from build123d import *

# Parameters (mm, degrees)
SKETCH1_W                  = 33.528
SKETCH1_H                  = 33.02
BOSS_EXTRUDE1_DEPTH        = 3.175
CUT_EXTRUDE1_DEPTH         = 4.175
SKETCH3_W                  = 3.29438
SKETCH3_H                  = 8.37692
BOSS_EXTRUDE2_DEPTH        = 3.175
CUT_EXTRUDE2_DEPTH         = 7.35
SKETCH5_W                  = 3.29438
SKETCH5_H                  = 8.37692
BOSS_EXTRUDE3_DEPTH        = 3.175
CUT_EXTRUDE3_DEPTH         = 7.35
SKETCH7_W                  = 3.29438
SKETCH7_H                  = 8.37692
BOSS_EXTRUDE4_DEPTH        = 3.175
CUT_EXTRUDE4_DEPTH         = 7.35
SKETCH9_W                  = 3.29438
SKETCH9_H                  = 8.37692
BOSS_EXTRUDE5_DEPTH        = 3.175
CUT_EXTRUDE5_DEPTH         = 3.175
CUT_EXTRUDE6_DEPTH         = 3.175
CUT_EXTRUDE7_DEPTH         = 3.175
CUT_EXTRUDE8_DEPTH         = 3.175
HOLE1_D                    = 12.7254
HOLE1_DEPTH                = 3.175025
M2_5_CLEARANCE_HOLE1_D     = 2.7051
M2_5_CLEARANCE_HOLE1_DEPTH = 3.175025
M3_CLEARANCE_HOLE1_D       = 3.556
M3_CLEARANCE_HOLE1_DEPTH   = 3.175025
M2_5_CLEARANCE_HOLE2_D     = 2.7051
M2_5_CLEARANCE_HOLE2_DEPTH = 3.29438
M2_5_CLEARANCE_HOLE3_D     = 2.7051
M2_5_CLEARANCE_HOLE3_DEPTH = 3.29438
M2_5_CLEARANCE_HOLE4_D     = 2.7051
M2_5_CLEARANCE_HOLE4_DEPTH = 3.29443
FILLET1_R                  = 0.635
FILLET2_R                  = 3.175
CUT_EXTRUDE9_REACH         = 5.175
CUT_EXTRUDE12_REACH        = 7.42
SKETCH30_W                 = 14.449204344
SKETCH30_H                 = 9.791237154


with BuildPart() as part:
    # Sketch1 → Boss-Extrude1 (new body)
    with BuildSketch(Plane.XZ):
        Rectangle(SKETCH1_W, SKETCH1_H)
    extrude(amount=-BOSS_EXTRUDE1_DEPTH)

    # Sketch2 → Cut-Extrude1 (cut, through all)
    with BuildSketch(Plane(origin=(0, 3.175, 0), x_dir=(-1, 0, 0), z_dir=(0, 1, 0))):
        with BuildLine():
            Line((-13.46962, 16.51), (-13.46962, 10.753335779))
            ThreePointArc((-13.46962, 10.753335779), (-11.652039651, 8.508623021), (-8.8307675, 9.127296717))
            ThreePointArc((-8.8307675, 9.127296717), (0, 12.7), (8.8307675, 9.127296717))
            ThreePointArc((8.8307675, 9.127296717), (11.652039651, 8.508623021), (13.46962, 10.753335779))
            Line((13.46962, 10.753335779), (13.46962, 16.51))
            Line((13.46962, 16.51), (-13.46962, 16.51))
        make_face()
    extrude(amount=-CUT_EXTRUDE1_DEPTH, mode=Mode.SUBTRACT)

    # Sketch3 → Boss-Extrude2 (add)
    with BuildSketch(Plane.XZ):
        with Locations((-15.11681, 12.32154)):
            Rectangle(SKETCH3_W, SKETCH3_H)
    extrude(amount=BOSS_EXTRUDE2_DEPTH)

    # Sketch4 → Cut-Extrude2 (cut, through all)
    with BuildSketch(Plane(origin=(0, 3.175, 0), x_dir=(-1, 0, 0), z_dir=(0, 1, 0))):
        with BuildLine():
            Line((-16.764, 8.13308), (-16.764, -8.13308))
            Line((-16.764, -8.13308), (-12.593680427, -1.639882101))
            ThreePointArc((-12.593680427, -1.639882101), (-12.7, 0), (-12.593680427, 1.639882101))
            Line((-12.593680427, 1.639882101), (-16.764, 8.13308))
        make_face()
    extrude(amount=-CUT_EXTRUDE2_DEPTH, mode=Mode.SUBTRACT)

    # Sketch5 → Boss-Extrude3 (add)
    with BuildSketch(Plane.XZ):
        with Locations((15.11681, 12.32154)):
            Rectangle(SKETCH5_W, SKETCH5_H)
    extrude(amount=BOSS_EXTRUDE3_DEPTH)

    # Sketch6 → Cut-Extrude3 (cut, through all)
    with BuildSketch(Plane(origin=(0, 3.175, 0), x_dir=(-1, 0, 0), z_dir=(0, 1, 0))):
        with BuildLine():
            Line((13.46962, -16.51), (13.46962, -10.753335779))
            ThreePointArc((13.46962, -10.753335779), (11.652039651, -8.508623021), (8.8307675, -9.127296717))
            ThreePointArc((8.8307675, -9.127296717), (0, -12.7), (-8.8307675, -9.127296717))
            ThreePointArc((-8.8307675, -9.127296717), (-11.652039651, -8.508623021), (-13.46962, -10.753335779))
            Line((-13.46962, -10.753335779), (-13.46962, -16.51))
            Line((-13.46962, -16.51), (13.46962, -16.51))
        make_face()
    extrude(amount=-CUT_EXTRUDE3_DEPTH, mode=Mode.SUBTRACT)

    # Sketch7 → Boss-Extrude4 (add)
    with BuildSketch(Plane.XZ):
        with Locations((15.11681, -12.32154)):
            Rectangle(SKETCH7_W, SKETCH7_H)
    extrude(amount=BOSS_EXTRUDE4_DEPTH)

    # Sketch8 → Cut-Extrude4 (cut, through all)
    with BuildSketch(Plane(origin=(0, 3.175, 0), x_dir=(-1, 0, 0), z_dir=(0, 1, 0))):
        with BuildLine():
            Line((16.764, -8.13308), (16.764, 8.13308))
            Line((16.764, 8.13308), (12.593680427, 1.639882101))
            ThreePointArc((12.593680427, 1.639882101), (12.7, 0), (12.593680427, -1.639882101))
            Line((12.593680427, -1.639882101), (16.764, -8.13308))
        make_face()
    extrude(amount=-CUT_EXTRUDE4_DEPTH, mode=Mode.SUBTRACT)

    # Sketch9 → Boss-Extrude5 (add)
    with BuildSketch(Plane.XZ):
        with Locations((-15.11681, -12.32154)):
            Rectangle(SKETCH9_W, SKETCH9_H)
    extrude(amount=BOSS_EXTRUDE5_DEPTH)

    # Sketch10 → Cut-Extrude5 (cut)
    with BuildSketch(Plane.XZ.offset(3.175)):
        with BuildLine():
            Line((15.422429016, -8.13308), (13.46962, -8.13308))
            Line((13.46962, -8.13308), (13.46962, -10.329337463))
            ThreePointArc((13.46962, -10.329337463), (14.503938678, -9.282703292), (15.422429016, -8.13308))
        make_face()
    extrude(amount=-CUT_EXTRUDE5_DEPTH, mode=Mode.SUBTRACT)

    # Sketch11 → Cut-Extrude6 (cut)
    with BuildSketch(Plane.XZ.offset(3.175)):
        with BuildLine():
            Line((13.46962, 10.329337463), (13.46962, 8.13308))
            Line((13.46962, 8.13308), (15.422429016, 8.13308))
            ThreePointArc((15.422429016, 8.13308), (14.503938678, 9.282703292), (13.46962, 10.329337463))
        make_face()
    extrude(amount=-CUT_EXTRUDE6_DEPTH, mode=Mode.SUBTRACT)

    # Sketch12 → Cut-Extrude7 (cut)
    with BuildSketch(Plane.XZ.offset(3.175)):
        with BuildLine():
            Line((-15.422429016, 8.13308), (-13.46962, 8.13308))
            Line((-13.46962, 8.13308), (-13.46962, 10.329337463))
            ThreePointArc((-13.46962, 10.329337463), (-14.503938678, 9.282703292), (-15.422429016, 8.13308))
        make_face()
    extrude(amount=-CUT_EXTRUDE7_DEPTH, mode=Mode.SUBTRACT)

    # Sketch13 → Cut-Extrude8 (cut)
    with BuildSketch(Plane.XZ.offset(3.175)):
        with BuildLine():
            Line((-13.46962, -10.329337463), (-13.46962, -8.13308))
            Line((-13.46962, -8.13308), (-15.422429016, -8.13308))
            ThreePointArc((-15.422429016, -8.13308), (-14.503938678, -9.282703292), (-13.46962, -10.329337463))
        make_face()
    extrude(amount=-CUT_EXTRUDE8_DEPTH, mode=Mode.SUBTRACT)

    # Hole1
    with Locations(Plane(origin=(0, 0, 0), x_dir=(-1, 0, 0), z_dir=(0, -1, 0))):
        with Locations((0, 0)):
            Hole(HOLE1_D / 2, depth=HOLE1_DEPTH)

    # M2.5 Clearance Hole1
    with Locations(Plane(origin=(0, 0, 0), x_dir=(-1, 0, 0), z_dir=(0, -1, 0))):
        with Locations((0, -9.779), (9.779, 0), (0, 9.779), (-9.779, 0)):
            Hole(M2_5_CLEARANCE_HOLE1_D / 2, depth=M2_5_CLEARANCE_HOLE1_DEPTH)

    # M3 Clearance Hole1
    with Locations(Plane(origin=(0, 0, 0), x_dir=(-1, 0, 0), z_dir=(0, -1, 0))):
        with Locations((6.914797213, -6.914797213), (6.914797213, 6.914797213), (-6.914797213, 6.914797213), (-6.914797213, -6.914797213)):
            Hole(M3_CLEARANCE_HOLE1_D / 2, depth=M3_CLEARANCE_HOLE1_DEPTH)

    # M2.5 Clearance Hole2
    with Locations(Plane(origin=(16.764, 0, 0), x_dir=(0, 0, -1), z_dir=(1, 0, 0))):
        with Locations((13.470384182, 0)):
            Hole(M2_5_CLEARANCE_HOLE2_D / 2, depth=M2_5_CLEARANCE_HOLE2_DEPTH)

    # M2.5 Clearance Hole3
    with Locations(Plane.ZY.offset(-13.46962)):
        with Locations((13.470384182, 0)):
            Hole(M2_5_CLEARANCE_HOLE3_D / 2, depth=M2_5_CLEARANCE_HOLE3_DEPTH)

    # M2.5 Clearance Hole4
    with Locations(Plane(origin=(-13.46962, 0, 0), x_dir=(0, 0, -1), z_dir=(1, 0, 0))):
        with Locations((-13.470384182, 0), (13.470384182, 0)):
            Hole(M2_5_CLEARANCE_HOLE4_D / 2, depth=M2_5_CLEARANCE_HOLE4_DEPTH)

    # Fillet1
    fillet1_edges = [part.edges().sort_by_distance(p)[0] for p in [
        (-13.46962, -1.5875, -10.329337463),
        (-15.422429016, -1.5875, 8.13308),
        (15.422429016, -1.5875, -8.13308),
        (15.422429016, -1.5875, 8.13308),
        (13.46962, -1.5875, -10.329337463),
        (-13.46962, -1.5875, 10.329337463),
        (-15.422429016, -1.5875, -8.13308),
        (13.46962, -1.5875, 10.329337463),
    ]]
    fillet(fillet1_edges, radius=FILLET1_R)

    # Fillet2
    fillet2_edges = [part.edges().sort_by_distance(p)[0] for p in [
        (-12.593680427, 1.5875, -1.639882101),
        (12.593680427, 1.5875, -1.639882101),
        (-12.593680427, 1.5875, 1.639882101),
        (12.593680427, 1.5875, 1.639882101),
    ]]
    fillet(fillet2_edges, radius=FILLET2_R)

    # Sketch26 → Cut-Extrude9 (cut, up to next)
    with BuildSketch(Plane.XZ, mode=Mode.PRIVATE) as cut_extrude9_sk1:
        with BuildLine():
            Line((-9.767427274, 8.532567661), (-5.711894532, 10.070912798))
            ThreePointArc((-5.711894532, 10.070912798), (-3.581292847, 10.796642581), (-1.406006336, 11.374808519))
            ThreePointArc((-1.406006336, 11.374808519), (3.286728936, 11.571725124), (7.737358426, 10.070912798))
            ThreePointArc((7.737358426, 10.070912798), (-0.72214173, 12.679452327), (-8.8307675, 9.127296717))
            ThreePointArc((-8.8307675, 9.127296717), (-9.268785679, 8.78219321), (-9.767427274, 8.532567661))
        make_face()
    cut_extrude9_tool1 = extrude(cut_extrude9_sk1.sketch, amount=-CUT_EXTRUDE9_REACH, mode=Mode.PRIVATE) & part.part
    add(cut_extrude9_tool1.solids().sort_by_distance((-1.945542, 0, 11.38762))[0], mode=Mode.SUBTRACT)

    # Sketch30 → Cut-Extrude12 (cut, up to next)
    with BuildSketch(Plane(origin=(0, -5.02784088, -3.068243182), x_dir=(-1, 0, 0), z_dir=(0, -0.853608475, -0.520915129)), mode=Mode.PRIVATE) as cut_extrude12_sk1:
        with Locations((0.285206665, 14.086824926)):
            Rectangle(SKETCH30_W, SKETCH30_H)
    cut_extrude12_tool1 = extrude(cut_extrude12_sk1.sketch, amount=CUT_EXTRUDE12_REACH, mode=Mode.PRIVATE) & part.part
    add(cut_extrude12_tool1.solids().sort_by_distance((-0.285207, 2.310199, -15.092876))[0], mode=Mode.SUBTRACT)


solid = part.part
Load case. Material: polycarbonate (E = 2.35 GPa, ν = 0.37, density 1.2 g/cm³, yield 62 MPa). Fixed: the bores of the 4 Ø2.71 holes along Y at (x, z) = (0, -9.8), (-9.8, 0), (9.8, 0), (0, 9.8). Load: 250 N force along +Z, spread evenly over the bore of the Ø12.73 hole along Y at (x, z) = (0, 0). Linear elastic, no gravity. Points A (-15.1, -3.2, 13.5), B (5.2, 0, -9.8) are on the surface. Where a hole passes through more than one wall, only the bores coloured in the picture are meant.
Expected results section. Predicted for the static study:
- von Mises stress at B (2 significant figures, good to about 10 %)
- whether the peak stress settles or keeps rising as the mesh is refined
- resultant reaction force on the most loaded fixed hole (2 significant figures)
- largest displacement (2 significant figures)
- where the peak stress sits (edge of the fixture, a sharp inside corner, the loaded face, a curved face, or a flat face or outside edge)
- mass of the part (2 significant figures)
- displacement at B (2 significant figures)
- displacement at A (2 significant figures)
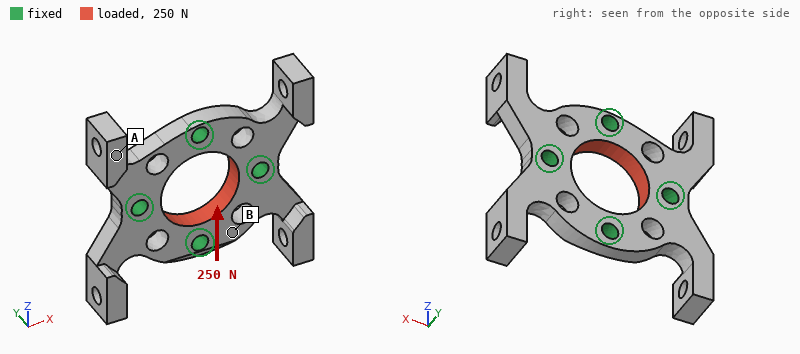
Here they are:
1.5 MPa
keeps rising
64 N
14 µm
edge of the fixture
2.2 g
6.2 µm
11 µm
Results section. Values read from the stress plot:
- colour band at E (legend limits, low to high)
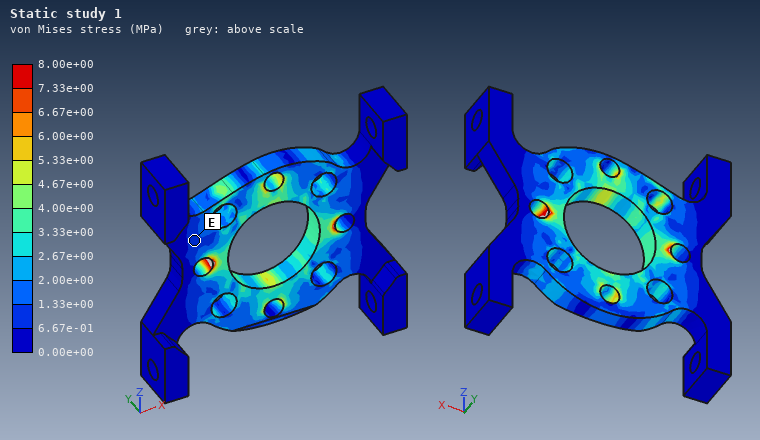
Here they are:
6.67e-01 to 1.33e+00 MPa
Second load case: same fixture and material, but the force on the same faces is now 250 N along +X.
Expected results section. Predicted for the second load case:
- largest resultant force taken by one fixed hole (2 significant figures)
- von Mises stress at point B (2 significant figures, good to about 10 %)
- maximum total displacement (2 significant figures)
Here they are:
63 N
1.6 MPa
14 µm
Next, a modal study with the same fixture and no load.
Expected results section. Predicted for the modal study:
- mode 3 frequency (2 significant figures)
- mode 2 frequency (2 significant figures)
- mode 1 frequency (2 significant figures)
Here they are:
2500 Hz
2500 Hz
2500 Hz
